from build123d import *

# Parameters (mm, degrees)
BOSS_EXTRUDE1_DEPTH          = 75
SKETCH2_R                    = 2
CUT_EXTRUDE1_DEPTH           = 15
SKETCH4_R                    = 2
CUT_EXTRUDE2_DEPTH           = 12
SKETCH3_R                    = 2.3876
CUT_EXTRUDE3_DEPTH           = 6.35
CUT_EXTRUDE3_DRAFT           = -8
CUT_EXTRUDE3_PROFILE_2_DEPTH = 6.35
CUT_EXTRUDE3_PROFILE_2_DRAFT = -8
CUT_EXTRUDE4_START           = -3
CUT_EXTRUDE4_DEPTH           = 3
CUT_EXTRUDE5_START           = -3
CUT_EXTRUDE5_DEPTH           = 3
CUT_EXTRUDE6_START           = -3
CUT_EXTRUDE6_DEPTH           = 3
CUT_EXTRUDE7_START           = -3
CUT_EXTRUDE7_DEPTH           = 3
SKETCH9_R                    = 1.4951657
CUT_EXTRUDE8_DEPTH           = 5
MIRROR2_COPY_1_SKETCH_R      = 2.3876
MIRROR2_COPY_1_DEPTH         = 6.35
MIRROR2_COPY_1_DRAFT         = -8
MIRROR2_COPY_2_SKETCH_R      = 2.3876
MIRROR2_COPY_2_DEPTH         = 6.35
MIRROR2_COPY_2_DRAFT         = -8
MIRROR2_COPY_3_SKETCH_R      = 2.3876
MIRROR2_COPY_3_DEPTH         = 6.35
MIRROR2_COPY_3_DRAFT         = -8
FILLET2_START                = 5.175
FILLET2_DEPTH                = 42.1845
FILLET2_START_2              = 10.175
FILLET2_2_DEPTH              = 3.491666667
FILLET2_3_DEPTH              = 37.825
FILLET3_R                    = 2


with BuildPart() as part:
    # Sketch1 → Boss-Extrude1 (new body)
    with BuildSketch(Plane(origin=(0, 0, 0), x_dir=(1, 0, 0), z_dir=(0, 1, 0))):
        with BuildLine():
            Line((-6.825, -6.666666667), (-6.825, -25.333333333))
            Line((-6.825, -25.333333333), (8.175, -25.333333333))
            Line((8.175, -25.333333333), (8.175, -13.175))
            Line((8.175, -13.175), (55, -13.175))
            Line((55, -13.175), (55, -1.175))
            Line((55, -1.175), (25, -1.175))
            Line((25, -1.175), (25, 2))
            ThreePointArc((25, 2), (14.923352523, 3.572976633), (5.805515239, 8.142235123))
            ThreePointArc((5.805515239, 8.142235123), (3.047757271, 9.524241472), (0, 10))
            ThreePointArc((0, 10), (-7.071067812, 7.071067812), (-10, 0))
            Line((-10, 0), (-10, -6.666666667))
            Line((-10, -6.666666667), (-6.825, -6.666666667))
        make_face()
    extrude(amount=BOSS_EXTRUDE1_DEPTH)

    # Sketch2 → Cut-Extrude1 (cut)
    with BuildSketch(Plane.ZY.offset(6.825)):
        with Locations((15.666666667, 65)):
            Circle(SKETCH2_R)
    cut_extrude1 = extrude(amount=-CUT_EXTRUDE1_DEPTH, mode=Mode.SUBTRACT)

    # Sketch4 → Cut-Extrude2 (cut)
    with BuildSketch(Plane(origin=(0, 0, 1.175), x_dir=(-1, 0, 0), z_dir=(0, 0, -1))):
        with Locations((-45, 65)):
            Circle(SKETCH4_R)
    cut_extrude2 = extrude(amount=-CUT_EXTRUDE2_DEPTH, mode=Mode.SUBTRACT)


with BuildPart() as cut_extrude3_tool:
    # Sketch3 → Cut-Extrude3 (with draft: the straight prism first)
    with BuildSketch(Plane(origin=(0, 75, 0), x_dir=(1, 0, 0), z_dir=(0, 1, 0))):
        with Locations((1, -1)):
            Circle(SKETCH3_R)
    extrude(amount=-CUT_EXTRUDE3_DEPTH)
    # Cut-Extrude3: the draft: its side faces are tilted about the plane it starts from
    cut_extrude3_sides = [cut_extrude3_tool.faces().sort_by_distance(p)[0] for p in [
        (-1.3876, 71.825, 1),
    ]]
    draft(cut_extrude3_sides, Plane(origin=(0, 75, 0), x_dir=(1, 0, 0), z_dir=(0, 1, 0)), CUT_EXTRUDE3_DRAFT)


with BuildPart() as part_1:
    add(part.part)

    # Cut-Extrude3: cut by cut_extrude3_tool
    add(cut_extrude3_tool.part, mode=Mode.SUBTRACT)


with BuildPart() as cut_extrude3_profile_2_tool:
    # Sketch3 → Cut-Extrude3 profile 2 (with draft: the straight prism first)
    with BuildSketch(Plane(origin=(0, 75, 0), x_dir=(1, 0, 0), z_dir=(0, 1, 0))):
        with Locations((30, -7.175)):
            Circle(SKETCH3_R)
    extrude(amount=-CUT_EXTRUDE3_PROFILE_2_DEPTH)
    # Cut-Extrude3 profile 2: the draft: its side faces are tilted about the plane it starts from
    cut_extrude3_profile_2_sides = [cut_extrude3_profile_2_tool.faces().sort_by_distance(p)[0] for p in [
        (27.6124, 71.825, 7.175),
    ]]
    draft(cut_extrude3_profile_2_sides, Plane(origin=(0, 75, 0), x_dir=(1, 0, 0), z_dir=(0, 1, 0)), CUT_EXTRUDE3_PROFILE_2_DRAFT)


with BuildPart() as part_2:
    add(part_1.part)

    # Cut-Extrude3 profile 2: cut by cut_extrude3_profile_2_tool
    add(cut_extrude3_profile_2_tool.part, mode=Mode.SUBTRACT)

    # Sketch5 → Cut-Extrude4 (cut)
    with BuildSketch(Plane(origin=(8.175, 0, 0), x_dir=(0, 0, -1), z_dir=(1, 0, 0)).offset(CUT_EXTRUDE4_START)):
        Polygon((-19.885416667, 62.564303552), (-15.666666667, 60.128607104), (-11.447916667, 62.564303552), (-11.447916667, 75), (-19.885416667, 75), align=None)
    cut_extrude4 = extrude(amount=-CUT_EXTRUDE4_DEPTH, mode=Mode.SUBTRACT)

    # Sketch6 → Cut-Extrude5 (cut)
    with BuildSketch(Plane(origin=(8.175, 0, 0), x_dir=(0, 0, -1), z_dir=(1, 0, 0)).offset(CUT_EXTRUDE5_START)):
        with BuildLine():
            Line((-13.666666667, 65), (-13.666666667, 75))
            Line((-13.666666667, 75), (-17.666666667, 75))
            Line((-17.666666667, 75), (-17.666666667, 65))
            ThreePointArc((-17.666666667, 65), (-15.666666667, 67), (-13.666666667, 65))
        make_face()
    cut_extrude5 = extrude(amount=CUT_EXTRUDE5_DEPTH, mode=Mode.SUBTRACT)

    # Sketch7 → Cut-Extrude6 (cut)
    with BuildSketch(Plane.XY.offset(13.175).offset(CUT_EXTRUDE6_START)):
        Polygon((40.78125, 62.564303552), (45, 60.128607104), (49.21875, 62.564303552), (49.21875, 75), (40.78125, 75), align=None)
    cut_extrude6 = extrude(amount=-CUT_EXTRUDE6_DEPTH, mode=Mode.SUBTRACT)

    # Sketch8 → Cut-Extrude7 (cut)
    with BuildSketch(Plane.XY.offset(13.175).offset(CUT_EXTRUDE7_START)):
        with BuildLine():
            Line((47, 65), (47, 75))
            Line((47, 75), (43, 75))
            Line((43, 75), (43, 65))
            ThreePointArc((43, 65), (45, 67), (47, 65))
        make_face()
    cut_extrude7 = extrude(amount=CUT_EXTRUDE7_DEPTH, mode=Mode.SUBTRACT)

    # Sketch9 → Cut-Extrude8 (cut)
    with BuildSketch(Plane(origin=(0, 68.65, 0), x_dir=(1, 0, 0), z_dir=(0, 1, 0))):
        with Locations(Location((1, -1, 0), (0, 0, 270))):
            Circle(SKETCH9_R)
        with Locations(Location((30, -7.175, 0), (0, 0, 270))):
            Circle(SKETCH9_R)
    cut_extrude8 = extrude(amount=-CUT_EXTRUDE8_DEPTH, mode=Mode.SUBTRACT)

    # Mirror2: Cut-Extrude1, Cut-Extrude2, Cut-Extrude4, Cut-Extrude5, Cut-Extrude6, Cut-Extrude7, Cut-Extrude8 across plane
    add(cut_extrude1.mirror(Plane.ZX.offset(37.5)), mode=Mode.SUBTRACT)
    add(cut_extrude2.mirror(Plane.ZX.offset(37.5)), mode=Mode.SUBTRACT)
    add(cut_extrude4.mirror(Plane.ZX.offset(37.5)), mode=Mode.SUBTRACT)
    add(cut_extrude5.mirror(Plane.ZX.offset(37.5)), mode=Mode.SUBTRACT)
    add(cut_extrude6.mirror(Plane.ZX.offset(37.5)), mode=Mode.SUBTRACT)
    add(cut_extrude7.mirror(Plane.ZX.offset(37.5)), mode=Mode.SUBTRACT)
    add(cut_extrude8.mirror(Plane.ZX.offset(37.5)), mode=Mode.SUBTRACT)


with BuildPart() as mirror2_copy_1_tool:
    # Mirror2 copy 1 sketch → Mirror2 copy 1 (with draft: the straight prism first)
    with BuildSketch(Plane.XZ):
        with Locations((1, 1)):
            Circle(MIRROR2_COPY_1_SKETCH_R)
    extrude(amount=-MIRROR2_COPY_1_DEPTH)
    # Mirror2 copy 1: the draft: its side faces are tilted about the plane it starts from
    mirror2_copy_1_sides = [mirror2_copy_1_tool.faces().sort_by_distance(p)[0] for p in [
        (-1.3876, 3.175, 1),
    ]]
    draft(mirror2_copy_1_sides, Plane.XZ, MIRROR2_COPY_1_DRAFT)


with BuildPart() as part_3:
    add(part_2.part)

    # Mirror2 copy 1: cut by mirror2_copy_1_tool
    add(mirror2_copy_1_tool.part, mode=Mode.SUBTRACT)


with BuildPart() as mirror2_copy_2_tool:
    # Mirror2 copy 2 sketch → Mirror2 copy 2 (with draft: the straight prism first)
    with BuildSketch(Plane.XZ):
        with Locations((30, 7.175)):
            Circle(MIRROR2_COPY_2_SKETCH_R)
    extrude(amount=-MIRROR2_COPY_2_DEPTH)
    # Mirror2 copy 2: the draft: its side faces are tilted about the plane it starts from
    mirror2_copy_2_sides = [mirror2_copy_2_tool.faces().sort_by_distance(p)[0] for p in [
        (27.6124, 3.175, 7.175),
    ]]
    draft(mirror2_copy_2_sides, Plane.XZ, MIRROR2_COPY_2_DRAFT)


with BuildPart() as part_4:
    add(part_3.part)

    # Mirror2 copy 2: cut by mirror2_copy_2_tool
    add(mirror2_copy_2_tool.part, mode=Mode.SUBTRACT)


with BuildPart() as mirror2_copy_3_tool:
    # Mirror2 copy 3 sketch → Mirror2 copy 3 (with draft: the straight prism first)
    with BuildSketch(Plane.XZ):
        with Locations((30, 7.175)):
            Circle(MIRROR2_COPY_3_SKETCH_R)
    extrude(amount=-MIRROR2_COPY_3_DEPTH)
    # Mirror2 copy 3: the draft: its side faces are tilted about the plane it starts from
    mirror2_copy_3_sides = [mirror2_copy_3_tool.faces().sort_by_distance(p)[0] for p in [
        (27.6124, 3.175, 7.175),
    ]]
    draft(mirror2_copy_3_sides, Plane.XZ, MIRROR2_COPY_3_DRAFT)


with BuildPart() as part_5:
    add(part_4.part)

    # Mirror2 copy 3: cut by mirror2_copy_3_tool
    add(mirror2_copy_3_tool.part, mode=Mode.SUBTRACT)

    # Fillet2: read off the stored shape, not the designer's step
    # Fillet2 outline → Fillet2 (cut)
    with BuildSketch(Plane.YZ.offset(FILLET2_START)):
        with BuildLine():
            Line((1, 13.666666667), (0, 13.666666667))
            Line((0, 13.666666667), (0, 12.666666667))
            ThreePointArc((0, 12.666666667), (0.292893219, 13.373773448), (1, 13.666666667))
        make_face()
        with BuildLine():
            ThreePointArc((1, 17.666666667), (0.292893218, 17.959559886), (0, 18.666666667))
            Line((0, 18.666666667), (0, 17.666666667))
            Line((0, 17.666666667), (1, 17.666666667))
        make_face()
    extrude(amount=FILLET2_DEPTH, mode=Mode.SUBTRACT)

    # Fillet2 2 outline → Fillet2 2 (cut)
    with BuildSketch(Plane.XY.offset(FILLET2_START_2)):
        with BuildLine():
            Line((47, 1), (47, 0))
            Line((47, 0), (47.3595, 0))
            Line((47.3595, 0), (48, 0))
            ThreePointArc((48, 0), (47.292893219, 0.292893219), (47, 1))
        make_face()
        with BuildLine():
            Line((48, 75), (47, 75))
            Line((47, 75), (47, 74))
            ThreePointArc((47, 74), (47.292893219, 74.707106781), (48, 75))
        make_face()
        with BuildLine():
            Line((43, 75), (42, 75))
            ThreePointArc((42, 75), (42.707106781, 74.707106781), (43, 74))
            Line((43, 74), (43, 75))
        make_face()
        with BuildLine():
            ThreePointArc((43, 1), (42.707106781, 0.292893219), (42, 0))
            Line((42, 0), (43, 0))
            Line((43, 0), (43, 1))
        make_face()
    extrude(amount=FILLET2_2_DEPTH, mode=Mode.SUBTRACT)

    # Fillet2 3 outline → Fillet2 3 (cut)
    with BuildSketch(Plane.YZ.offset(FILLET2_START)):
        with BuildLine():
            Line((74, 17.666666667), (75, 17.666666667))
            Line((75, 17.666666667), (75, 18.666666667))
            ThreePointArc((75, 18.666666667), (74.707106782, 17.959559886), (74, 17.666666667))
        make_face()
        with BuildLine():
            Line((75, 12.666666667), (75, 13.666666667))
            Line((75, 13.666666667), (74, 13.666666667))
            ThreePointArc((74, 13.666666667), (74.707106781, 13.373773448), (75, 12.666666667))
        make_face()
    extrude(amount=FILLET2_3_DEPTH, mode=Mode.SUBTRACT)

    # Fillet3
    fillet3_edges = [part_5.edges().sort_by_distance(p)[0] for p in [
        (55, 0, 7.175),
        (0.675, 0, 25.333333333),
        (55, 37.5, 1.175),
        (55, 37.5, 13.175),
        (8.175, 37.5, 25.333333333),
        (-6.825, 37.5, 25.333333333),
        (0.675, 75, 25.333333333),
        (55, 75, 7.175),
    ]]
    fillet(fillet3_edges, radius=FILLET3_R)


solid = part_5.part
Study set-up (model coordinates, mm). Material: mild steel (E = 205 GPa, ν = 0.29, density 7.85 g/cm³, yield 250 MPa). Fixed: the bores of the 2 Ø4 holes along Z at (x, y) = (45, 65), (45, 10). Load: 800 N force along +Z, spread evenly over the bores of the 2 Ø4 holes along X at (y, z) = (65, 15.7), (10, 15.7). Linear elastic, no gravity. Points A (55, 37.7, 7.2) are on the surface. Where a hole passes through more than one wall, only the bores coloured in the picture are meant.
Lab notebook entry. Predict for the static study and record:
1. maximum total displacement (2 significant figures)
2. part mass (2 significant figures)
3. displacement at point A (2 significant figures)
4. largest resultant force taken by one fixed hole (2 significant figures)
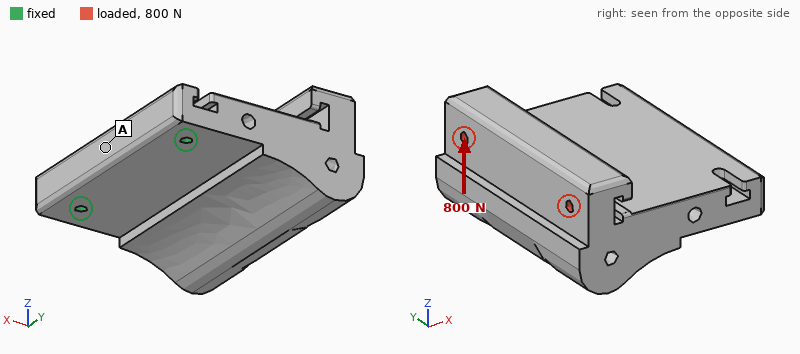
62 µm
680 g
9.4 µm
410 N
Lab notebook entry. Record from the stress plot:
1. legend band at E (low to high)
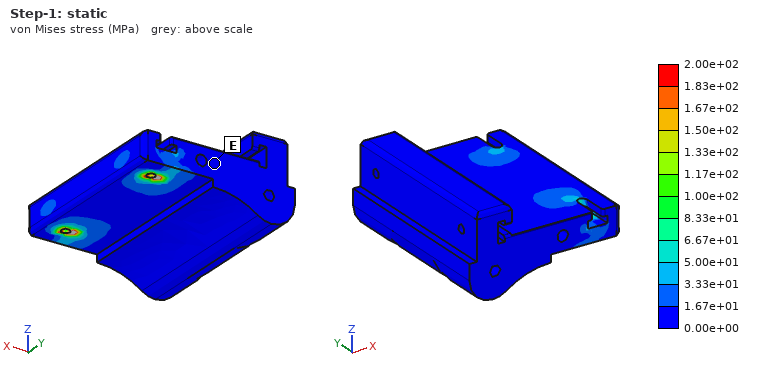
0.00e+00 to 1.67e+01 MPa
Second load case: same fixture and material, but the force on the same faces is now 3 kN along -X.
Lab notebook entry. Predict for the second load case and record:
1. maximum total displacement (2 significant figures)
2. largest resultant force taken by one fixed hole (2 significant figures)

60 µm
1.5 kN
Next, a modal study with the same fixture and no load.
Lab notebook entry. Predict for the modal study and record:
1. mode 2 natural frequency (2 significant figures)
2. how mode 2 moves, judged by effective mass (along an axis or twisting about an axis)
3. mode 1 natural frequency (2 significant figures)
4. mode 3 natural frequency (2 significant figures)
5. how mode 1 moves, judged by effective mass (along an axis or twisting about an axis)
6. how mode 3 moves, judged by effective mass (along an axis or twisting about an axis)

4200 Hz
twisting about X
1000 Hz
5900 Hz
along Z
along Y
